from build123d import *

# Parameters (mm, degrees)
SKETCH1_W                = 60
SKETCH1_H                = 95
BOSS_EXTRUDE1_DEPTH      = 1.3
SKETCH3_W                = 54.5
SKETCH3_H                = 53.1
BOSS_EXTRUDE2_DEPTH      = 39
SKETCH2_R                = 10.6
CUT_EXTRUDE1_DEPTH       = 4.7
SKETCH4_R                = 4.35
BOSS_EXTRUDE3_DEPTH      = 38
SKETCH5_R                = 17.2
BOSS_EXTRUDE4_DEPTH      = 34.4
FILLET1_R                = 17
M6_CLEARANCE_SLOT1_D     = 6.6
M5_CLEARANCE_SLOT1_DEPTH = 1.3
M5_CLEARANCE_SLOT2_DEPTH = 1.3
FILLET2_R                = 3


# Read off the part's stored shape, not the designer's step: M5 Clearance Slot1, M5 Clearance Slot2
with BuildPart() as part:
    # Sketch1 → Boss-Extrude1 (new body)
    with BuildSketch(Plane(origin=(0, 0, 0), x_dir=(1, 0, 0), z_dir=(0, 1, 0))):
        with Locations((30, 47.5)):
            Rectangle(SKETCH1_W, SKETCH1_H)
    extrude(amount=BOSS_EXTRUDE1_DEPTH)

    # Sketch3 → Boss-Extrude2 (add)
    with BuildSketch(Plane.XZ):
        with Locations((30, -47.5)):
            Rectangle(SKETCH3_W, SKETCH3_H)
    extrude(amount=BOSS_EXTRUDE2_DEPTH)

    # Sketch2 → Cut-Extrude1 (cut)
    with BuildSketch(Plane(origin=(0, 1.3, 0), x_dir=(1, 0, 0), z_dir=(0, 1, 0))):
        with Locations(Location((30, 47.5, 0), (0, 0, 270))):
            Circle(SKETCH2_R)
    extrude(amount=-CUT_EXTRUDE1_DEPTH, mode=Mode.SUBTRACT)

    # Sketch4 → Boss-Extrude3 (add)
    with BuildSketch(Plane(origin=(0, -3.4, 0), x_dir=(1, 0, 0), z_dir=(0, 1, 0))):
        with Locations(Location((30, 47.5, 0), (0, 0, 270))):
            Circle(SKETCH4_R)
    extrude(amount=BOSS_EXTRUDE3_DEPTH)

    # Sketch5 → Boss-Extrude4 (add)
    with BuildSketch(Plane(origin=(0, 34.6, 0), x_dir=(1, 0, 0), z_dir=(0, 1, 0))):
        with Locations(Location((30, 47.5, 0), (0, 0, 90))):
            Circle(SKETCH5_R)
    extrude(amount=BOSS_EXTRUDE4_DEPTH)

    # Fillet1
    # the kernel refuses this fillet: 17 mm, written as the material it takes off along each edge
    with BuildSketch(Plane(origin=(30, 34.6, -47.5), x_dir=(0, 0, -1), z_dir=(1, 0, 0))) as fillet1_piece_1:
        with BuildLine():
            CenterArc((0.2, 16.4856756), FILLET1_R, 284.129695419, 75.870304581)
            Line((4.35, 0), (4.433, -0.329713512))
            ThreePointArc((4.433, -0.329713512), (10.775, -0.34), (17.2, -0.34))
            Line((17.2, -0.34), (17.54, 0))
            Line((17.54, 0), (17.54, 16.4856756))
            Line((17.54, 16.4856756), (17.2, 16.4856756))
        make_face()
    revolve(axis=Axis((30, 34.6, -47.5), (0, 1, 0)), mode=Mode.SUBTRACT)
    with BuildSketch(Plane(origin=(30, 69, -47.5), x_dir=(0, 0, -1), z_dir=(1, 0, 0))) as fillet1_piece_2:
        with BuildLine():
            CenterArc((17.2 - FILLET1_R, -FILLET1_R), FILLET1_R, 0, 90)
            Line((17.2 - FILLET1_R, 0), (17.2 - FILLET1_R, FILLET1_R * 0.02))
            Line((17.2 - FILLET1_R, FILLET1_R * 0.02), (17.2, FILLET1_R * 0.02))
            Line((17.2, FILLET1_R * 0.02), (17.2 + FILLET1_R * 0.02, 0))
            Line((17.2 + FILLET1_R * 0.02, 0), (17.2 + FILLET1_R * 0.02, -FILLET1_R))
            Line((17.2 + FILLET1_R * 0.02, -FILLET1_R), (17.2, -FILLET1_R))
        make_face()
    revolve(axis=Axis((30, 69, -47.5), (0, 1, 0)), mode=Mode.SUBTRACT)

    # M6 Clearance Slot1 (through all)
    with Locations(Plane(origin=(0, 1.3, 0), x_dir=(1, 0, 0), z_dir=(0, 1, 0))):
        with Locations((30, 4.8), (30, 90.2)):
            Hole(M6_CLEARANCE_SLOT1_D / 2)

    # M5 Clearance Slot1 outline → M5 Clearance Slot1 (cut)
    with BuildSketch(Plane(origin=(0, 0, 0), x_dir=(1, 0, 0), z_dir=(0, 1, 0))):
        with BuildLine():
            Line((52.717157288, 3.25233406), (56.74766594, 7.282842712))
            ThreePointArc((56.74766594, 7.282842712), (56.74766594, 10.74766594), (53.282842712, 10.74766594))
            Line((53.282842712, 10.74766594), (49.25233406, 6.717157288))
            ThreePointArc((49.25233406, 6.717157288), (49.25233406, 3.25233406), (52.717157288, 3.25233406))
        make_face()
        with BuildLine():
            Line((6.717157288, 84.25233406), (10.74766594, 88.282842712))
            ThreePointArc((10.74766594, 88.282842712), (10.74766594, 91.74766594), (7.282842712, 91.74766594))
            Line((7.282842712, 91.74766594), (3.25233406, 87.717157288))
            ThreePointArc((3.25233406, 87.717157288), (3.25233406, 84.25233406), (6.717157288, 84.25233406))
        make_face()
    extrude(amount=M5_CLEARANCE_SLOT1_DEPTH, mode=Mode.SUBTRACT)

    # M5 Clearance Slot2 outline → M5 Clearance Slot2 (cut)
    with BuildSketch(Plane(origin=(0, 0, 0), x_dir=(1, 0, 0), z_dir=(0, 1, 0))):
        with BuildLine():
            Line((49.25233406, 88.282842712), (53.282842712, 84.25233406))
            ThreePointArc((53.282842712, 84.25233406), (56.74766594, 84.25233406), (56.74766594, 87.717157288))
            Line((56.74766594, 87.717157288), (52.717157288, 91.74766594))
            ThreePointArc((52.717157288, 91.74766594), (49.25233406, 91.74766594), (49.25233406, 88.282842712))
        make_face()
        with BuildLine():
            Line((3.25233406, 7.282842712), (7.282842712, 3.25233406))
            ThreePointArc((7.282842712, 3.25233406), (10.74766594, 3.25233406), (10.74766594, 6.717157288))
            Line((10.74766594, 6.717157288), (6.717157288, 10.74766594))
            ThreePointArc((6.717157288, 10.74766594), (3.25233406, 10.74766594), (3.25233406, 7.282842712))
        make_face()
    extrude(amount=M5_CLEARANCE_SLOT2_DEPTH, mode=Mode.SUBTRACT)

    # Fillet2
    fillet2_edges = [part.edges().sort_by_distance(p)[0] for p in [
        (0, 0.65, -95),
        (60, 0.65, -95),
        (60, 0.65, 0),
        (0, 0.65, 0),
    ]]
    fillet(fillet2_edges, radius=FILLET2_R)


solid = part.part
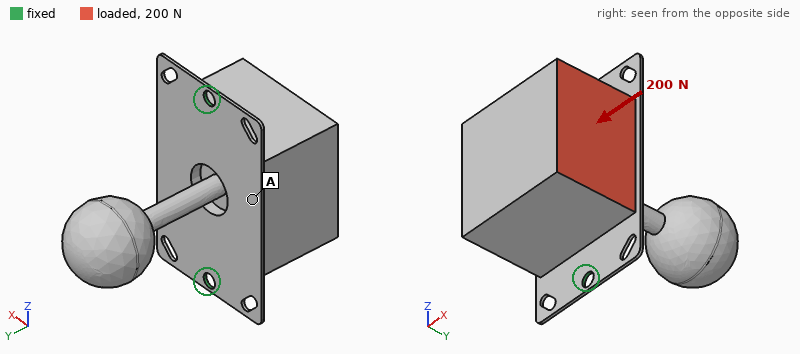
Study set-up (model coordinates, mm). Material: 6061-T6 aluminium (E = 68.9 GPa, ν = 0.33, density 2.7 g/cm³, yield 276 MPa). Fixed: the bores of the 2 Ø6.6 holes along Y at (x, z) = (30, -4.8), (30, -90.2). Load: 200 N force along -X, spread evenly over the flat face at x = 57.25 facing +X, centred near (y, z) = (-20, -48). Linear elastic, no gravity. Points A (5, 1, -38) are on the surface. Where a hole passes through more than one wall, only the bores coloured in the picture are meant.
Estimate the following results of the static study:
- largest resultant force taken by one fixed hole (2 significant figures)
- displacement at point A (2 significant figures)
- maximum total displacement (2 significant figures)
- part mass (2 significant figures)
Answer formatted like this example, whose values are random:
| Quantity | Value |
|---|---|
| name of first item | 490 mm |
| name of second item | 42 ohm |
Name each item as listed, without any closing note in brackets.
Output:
| Quantity | Value |
|---|---|
| largest resultant force taken by one fixed hole | 100 N |
| displacement at point A | 0.58 mm |
| maximum total displacement | 1.6 mm |
| part mass | 380 g |
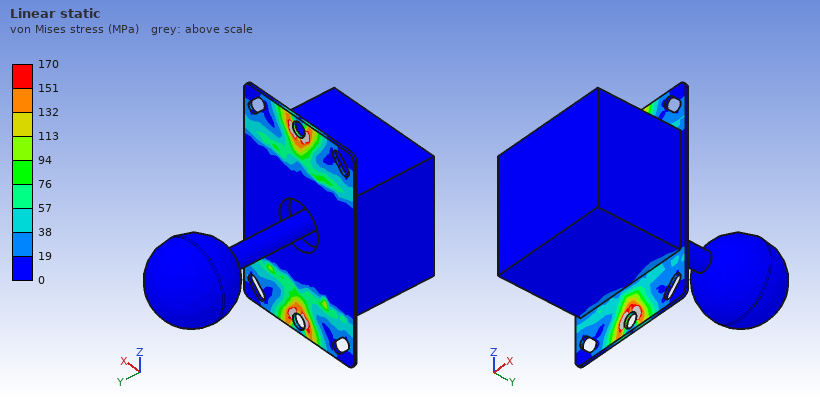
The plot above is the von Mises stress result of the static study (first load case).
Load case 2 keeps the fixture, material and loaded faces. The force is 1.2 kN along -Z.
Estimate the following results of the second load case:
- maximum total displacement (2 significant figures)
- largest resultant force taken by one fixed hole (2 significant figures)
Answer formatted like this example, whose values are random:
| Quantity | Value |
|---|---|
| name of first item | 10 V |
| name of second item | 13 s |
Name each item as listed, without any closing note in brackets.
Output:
| Quantity | Value |
|---|---|
| maximum total displacement | 0.48 mm |
| largest resultant force taken by one fixed hole | 790 N |
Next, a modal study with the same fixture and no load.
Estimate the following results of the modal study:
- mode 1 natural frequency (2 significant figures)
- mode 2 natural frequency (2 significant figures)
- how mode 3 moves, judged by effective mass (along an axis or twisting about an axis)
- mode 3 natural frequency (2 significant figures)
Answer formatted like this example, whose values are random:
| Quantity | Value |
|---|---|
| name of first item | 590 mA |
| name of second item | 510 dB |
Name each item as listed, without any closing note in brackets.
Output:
| Quantity | Value |
|---|---|
| mode 1 natural frequency | 100 Hz |
| mode 2 natural frequency | 310 Hz |
| how mode 3 moves, judged by effective mass | along Y |
| mode 3 natural frequency | 430 Hz |
